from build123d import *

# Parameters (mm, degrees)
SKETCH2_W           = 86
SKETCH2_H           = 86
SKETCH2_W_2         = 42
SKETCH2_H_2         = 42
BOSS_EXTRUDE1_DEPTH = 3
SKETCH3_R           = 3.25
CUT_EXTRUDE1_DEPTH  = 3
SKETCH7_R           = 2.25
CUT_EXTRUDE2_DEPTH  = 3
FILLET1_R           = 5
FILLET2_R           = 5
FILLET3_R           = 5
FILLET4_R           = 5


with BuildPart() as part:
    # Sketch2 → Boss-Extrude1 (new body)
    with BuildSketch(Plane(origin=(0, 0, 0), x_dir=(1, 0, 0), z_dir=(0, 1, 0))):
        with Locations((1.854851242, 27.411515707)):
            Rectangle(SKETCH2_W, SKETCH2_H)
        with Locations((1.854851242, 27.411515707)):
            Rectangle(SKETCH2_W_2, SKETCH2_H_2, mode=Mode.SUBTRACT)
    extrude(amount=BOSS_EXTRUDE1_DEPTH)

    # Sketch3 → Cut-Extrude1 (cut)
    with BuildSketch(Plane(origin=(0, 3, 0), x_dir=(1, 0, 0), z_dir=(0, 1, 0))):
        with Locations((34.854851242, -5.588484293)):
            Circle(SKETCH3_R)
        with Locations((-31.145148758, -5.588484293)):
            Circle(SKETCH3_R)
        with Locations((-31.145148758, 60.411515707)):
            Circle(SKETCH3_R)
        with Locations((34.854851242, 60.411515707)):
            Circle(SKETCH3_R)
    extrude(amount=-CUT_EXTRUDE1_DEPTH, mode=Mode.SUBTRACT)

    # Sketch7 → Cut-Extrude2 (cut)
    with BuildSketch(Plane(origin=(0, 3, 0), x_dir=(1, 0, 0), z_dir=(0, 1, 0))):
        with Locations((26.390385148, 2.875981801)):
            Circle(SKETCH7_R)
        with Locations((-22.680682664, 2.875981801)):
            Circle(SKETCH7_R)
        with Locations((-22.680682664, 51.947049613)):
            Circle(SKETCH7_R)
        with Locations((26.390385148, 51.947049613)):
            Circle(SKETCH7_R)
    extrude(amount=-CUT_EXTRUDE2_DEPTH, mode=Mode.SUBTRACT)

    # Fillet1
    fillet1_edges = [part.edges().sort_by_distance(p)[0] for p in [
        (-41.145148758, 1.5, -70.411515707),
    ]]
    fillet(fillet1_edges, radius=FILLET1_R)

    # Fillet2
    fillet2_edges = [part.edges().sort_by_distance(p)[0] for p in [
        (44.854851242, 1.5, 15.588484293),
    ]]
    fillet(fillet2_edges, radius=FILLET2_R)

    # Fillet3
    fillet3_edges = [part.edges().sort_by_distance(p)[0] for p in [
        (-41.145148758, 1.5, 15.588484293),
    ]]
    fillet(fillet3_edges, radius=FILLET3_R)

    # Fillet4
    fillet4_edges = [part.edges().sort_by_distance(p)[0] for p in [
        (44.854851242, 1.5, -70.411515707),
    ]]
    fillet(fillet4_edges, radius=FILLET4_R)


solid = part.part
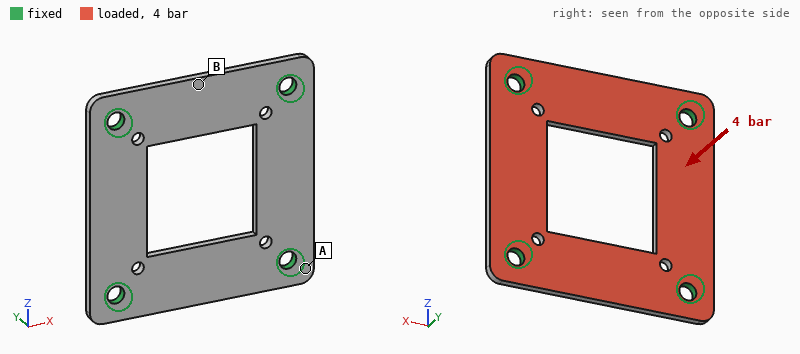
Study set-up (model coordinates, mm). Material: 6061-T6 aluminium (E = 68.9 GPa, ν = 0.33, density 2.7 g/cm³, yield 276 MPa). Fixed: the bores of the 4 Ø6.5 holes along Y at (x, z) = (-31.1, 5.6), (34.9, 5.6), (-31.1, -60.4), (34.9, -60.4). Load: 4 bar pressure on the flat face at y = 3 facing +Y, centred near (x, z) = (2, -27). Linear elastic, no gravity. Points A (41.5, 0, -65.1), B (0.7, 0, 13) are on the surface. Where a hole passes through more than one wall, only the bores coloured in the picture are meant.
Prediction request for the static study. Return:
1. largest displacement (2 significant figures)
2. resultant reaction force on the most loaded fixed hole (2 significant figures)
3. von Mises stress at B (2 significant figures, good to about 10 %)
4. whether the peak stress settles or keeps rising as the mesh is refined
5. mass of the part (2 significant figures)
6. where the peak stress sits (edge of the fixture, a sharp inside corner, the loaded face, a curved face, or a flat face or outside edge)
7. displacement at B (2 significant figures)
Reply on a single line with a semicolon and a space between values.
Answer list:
0.13 mm; 540 N; 40 MPa; keeps rising; 44 g; edge of the fixture; 0.092 mm
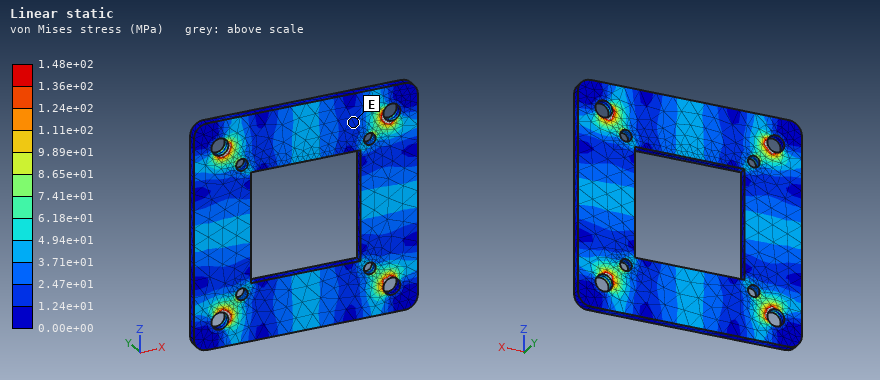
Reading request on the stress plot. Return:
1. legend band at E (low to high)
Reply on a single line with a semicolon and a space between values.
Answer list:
1.24e+01 to 2.47e+01 MPa
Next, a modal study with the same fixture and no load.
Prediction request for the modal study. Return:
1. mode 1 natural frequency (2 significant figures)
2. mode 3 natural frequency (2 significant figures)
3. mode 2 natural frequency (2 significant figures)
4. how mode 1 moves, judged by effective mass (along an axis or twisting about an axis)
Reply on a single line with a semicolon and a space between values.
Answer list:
3800 Hz; 4000 Hz; 4000 Hz; along Y
